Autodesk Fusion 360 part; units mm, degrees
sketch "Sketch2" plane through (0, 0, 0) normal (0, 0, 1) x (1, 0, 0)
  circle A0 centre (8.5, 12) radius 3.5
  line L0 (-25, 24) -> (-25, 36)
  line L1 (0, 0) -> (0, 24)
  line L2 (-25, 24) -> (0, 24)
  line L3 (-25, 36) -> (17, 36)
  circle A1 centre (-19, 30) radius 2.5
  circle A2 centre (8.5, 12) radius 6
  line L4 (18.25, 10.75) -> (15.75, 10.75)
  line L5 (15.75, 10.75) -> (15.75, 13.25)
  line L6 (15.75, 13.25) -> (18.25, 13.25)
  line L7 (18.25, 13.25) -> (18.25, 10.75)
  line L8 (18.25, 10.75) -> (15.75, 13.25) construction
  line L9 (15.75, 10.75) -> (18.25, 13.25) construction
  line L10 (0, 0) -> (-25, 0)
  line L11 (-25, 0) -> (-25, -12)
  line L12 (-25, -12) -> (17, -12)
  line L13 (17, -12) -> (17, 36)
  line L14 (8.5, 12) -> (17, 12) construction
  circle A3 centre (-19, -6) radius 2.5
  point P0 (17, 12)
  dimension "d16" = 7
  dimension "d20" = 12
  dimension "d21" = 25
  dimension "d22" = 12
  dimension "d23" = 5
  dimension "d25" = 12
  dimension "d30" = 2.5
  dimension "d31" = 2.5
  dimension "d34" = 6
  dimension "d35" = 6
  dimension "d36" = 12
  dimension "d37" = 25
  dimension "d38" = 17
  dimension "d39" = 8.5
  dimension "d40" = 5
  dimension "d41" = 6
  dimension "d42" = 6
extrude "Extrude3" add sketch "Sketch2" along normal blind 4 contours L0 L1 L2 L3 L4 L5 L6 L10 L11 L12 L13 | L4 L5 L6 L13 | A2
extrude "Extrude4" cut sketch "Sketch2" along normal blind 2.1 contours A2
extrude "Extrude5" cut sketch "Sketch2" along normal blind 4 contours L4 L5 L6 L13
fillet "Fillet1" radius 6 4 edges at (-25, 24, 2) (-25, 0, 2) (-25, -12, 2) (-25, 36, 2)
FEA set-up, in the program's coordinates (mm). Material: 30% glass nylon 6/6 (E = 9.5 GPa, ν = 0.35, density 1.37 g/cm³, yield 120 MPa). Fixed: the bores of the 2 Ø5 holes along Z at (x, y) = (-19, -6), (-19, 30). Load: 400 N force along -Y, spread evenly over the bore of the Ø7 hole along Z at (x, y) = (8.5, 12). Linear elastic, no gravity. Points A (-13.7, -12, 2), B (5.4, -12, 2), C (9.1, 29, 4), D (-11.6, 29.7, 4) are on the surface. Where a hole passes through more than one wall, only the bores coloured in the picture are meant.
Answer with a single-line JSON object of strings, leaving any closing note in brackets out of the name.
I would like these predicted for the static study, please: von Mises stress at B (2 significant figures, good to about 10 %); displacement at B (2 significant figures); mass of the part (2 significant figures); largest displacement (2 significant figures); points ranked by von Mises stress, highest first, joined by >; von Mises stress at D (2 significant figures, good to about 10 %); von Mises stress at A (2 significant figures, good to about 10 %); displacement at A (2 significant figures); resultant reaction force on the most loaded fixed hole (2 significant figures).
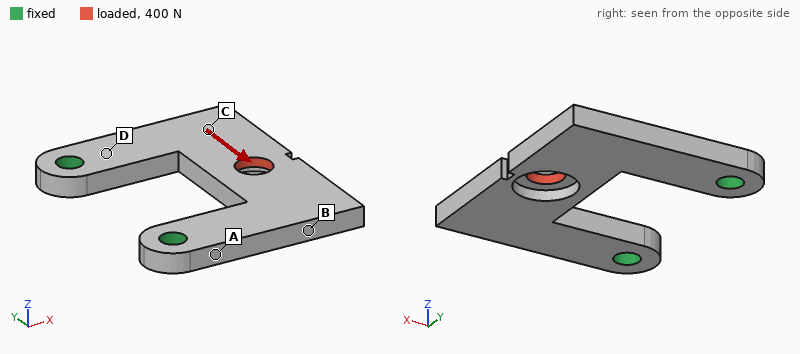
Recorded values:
{"von Mises stress at B": "7.5 MPa", "displacement at B": "0.11 mm", "mass of the part": "6.9 g", "largest displacement": "0.14 mm", "points ranked by von Mises stress, highest first, joined by >": "A > D > B > C", "von Mises stress at D": "12 MPa", "von Mises stress at A": "18 MPa", "displacement at A": "0.028 mm", "resultant reaction force on the most loaded fixed hole": "260 N"}
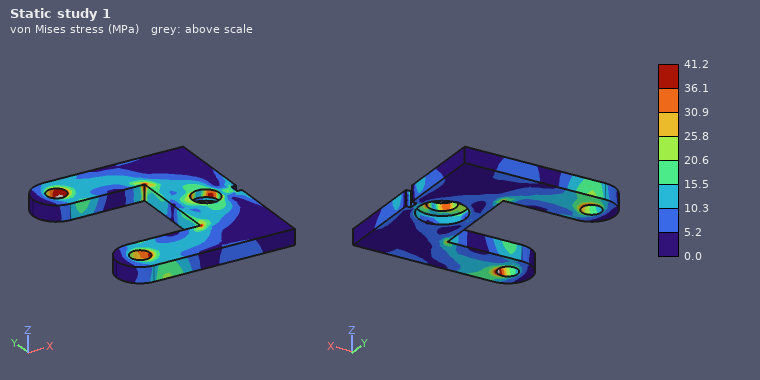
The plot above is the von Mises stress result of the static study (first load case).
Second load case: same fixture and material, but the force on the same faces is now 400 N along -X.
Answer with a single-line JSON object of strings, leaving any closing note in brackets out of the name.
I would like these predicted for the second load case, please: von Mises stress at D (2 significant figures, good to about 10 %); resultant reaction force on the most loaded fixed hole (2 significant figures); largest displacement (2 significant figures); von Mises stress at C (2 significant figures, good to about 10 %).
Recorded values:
{"von Mises stress at D": "12 MPa", "resultant reaction force on the most loaded fixed hole": "210 N", "largest displacement": "0.22 mm", "von Mises stress at C": "5.0 MPa"}
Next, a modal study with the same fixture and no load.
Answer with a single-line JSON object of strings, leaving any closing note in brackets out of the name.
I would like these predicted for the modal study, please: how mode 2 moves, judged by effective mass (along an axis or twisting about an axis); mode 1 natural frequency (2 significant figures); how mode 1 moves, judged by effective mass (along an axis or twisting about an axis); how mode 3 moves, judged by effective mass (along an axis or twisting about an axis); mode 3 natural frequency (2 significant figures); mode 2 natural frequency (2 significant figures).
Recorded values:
{"how mode 2 moves, judged by effective mass": "twisting about X", "mode 1 natural frequency": "1100 Hz", "how mode 1 moves, judged by effective mass": "along Z", "how mode 3 moves, judged by effective mass": "along Y", "mode 3 natural frequency": "4400 Hz", "mode 2 natural frequency": "2200 Hz"}
